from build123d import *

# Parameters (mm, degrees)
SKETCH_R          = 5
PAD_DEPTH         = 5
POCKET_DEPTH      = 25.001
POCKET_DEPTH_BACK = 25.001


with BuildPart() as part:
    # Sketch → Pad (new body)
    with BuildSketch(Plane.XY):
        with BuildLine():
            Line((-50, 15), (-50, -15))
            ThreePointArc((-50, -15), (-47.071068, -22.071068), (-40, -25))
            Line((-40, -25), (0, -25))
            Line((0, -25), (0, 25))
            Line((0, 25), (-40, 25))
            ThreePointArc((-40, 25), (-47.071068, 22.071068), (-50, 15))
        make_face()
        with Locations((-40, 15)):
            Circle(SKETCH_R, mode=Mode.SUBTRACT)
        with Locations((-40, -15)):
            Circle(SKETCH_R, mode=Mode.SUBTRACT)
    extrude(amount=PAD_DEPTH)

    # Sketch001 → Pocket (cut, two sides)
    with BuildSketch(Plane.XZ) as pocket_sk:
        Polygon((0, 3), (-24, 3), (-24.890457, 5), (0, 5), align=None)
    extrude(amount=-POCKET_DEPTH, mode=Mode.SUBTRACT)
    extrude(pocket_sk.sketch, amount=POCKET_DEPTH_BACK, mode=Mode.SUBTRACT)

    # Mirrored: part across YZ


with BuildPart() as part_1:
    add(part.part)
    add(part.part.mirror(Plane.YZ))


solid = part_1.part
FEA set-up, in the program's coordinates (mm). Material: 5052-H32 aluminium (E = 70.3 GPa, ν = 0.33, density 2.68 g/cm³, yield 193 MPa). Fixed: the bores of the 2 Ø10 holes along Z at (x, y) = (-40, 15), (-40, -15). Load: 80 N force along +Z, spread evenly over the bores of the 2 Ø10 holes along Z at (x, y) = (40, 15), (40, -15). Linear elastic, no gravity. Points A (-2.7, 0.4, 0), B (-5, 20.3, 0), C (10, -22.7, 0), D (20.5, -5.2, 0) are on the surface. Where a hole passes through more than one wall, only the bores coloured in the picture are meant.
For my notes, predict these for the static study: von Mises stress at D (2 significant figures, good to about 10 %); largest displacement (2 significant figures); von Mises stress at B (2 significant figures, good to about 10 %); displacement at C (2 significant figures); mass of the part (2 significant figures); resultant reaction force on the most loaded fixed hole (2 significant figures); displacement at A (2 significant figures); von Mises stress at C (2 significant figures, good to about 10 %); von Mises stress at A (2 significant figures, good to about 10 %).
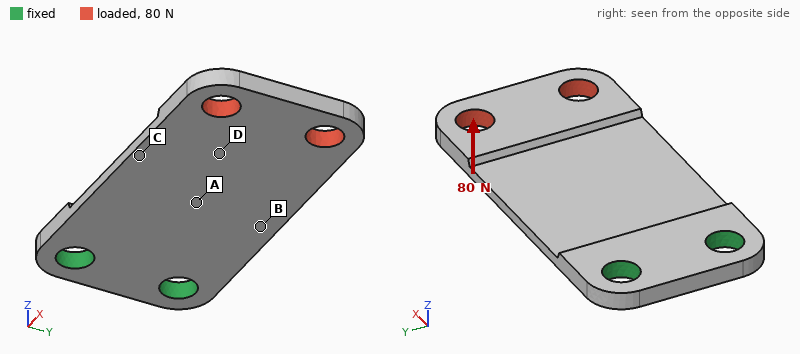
20 MPa
1.2 mm
48 MPa
0.38 mm
49 g
42 N
0.20 mm
34 MPa
40 MPa
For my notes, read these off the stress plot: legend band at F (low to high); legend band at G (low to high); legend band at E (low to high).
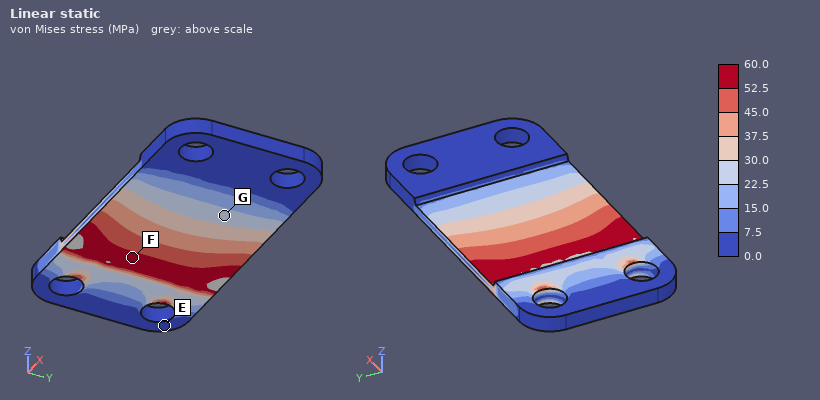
52.5 to 60.0 MPa
22.5 to 30.0 MPa
0.0 to 7.5 MPa
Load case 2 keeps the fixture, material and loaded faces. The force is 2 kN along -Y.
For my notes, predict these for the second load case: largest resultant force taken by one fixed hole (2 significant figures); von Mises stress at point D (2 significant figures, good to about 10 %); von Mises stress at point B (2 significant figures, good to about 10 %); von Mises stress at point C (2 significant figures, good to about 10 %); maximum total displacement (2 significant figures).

4.5 kN
26 MPa
57 MPa
34 MPa
0.28 mm
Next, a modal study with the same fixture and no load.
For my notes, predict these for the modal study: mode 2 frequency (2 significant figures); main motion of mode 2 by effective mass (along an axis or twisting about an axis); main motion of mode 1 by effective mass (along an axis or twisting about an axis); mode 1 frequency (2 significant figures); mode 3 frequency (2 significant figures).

1400 Hz
twisting about X
along Z
370 Hz
2500 Hz
